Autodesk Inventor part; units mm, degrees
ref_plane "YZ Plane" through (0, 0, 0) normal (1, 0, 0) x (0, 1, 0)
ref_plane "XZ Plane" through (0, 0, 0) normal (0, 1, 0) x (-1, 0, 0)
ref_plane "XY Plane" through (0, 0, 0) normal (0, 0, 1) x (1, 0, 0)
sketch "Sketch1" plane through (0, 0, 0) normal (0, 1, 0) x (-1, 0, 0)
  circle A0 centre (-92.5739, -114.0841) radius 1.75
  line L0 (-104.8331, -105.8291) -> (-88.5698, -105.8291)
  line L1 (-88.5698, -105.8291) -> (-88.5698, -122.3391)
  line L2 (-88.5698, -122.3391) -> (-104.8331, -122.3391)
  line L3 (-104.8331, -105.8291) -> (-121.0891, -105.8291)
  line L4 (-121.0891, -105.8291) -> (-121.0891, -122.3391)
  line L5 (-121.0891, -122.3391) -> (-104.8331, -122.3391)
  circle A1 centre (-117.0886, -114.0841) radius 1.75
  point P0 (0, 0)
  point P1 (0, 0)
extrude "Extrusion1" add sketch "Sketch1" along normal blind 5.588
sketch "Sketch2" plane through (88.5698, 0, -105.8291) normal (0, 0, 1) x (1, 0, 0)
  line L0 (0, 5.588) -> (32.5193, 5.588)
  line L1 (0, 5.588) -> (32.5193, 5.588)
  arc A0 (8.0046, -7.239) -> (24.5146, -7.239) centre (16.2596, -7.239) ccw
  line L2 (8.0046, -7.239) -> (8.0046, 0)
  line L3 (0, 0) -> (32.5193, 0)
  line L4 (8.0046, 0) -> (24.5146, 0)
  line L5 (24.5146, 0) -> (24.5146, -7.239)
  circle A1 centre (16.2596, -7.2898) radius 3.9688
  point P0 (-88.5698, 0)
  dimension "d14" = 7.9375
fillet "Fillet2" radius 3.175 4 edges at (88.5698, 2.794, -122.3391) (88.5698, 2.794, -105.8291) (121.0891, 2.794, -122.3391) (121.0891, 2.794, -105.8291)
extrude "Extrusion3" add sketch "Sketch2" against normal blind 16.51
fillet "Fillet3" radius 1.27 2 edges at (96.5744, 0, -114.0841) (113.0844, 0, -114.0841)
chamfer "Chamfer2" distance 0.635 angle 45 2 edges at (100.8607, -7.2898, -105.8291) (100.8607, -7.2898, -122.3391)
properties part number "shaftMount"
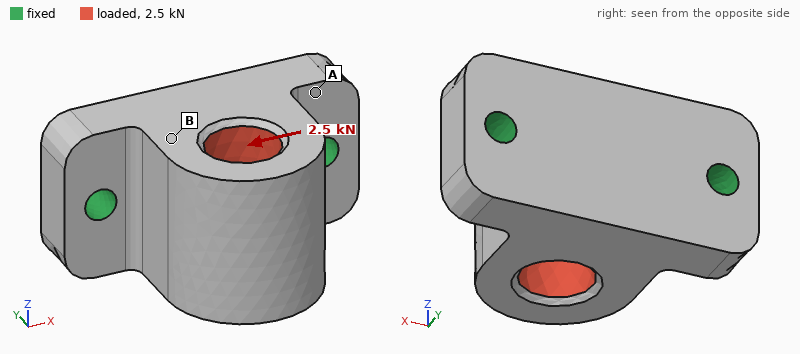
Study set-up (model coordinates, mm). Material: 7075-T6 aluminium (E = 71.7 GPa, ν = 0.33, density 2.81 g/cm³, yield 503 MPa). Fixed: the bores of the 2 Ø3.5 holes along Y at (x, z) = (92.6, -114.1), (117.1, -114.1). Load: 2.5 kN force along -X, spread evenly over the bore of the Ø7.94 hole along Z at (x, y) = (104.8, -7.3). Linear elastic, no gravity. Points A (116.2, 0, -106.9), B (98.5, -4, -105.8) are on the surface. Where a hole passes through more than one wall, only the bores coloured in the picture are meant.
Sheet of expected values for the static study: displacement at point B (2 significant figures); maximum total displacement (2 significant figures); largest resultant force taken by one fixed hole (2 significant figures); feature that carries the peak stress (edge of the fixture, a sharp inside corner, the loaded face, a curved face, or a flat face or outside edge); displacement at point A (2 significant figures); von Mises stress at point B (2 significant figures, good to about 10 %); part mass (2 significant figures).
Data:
6.8 µm
19 µm
1.7 kN
a curved face
3.3 µm
18 MPa
16 g
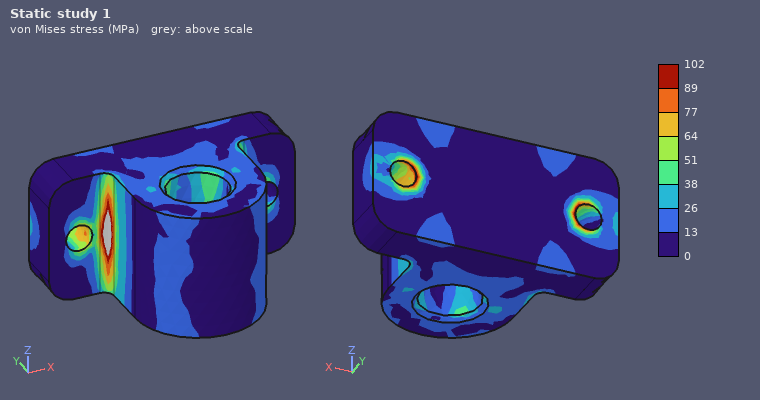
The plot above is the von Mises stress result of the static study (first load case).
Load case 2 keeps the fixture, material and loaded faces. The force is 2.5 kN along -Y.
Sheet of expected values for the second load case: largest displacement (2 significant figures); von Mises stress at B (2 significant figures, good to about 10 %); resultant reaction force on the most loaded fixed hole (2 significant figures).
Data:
8.2 µm
11 MPa
1.3 kN
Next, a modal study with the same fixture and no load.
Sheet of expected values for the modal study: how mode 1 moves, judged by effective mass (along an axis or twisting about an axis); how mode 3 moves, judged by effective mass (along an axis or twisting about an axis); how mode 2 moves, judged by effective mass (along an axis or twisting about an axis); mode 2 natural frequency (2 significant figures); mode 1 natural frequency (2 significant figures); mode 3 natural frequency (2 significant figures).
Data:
along Z
along Y
along X
23 kHz
12 kHz
27 kHz
